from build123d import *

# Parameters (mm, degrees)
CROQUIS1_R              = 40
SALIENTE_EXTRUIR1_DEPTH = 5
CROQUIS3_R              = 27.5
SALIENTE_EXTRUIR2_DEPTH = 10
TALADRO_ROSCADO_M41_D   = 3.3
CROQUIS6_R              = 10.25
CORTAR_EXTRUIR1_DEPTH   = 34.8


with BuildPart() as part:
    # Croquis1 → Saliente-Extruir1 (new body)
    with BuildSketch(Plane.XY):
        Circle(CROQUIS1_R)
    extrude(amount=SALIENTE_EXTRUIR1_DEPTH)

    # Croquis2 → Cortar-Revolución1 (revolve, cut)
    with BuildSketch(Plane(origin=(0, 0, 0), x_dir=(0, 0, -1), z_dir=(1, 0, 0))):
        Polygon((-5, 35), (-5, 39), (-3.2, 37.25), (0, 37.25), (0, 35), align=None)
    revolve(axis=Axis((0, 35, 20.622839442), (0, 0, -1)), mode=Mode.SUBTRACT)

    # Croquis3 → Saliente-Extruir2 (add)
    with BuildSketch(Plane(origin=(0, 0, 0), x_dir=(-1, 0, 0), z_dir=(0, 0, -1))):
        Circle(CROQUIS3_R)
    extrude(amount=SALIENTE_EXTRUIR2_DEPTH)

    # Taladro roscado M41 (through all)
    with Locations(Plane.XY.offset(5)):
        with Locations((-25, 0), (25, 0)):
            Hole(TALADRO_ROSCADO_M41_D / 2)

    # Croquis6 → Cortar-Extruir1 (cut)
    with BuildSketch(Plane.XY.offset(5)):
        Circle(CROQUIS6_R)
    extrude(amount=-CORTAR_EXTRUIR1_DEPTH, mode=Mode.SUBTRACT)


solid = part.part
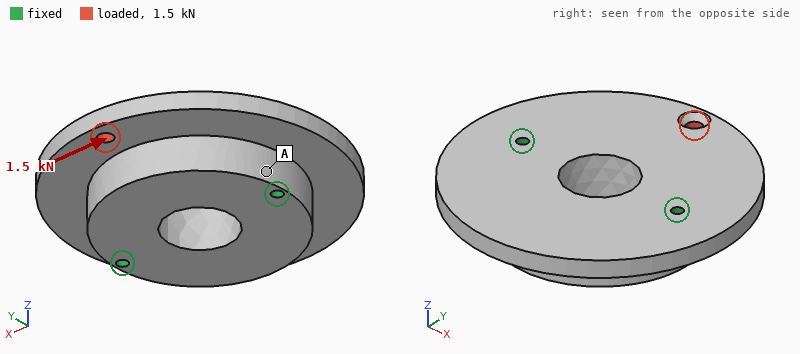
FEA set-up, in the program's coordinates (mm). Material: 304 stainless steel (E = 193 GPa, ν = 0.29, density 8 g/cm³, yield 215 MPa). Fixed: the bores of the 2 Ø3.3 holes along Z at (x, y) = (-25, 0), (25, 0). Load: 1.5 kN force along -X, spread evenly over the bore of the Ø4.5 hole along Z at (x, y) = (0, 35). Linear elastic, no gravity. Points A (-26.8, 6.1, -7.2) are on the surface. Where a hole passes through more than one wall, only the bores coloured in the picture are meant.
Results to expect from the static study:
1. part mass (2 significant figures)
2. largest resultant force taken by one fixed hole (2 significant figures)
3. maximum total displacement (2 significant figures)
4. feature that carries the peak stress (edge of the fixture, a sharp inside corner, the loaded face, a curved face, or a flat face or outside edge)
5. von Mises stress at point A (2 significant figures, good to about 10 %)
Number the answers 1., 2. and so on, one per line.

1. 350 g
2. 1.3 kN
3. 3.8 µm
4. the loaded face
5. 5.4 MPa
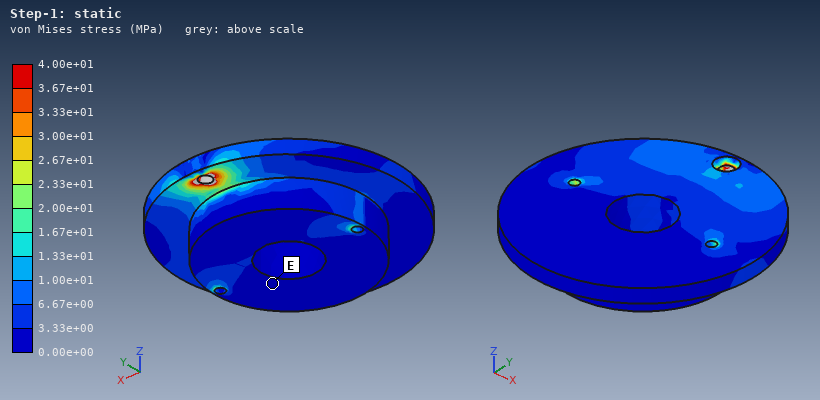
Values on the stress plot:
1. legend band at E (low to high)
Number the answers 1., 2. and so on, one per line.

1. 0.00e+00 to 3.33e+00 MPa
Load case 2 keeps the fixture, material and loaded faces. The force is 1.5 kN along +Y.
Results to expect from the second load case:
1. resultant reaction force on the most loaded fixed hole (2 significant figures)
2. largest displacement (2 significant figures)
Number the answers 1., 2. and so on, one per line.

1. 810 N
2. 4.2 µm
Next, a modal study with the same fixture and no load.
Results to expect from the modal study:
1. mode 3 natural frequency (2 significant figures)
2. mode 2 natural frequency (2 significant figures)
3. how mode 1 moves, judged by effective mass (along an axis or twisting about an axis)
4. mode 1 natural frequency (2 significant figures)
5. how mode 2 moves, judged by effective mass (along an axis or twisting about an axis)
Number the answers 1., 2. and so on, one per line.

1. 12 kHz
2. 8000 Hz
3. twisting about X
4. 6100 Hz
5. along Z
